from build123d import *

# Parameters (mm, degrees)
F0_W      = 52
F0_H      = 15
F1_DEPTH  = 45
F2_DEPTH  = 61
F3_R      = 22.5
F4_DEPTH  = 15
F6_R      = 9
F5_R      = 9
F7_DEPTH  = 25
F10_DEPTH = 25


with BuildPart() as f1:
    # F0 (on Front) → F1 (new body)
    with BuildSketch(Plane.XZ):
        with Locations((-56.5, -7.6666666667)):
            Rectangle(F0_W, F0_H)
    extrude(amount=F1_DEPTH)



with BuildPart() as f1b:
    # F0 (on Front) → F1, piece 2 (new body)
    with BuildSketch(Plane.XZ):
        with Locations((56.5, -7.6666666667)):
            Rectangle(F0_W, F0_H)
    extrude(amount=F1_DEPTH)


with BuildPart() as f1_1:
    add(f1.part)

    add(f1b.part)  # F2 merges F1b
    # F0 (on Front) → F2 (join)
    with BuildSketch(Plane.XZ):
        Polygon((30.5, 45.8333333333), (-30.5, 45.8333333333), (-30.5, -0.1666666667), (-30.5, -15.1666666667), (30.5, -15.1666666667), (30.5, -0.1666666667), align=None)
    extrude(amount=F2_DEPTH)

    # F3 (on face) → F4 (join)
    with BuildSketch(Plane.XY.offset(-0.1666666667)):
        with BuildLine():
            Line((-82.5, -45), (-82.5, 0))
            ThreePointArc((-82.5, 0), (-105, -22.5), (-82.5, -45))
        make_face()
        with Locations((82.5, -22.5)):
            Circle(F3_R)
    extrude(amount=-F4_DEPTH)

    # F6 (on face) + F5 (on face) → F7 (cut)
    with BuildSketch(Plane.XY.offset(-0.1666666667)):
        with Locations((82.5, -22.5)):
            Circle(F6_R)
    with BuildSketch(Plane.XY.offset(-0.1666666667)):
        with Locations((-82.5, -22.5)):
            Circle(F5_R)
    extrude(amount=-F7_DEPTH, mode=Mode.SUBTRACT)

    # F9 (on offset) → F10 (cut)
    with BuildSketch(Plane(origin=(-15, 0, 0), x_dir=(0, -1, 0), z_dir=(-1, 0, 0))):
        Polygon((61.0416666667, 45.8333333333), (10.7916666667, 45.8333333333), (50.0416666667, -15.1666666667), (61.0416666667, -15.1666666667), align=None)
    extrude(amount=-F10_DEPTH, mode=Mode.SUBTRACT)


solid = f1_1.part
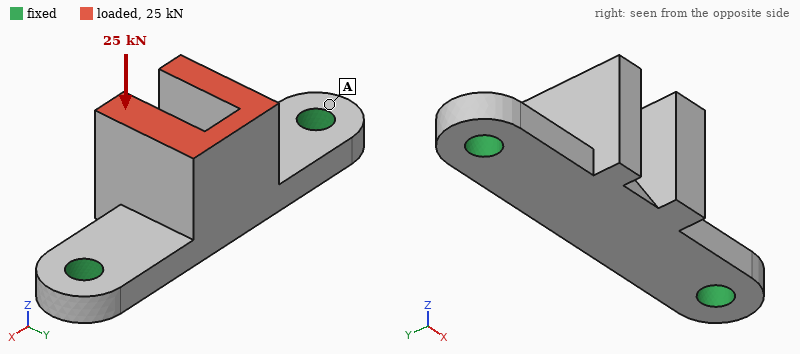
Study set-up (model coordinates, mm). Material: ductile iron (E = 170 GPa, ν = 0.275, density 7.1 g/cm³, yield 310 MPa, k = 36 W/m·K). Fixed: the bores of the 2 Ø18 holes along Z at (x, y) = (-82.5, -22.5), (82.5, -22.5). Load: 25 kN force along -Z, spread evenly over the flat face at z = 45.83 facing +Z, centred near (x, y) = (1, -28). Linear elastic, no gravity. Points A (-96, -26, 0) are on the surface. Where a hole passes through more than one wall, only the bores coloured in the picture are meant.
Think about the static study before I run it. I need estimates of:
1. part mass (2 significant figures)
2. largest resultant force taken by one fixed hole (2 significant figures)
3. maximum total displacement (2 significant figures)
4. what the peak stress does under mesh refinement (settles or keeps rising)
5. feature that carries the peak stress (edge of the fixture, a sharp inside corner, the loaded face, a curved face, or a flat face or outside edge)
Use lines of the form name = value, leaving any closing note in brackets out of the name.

part mass = 1.9 kg
largest resultant force taken by one fixed hole = 14 kN
maximum total displacement = 0.15 mm
what the peak stress does under mesh refinement = keeps rising
feature that carries the peak stress = edge of the fixture
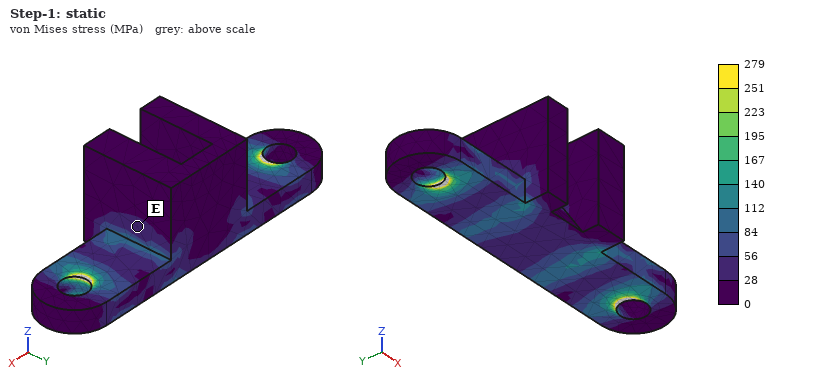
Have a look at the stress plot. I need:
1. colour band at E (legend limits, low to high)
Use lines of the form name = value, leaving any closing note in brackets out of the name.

colour band at E = 28 to 56 MPa
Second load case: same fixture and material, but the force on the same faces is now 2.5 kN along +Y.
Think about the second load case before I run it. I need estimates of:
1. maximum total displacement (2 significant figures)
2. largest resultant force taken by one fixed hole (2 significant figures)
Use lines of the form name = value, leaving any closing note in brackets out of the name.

maximum total displacement = 77 µm
largest resultant force taken by one fixed hole = 1.3 kN
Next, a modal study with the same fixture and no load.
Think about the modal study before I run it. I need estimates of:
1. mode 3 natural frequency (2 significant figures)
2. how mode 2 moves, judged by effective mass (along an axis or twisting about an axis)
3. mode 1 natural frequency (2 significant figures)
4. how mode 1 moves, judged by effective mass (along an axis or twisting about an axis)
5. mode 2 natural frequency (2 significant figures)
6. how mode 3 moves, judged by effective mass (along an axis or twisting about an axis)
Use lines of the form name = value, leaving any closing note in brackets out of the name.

mode 3 natural frequency = 3400 Hz
how mode 2 moves, judged by effective mass = along Z
mode 1 natural frequency = 1400 Hz
how mode 1 moves, judged by effective mass = along Y
mode 2 natural frequency = 2200 Hz
how mode 3 moves, judged by effective mass = along X
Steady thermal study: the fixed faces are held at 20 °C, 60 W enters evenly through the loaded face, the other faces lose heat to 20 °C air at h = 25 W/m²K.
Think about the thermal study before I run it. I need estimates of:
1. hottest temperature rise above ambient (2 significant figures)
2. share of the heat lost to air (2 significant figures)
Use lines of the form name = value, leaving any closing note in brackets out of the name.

hottest temperature rise above ambient = 64 K
share of the heat lost to air = 48 %
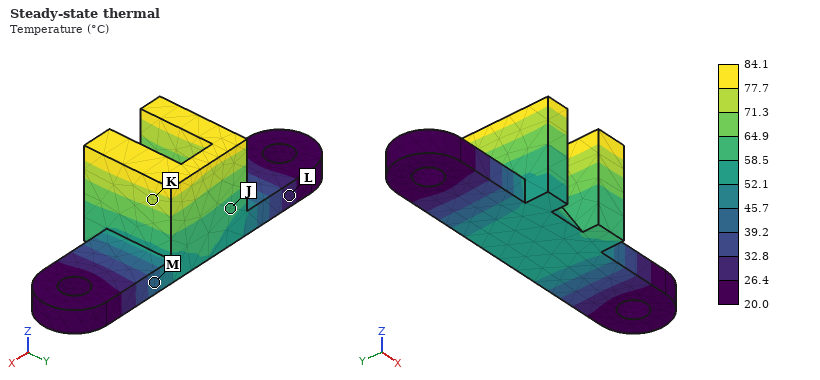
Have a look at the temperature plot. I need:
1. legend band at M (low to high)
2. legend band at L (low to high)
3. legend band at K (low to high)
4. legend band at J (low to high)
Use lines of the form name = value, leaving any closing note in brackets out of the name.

legend band at M = 39.2 to 45.7 °C
legend band at L = 26.4 to 32.8 °C
legend band at K = 71.3 to 77.7 °C
legend band at J = 58.5 to 64.9 °C
